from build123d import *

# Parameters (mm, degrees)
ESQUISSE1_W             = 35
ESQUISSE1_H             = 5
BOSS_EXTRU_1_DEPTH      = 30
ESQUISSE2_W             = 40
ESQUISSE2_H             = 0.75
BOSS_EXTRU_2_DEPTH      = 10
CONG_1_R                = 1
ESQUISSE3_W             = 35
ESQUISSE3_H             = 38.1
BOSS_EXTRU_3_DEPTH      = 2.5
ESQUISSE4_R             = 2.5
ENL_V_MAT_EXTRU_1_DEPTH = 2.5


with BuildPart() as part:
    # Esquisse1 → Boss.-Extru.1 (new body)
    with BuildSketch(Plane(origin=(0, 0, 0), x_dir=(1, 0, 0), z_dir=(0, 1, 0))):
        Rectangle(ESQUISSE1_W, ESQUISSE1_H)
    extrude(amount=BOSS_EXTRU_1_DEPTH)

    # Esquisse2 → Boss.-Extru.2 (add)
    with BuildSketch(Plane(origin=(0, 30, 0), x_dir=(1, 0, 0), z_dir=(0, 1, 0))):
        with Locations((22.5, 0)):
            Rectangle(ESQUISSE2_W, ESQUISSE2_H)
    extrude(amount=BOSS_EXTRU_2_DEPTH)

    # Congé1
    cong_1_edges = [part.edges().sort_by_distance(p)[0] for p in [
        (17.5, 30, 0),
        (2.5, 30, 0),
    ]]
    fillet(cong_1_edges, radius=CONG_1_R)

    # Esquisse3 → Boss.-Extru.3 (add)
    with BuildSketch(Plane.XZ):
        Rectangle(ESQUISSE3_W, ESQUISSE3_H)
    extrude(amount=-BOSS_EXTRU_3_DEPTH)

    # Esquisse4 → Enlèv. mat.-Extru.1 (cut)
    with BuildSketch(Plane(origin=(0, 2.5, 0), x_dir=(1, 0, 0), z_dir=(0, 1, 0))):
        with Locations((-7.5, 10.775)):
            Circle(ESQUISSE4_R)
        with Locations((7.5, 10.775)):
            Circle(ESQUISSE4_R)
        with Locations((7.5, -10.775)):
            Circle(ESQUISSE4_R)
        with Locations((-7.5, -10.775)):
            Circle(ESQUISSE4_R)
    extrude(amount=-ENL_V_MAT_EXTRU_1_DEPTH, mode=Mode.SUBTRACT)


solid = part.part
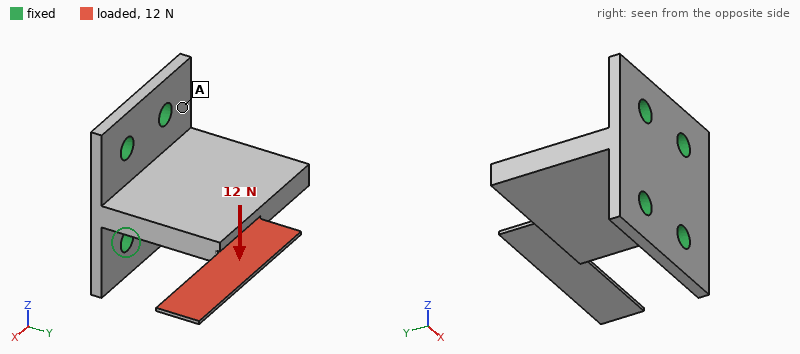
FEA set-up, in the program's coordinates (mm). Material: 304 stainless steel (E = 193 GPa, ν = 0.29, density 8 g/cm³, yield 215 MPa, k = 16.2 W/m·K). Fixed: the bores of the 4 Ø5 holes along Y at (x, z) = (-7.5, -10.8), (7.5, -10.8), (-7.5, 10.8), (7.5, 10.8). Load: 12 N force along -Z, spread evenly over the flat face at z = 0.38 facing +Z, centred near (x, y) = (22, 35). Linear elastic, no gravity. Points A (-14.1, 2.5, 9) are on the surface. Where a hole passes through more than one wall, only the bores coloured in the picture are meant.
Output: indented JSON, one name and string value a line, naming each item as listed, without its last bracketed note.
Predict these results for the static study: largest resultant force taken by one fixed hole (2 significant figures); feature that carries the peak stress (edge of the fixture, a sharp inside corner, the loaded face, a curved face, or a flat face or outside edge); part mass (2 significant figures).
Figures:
{
  "largest resultant force taken by one fixed hole": "20 N",
  "feature that carries the peak stress": "the loaded face",
  "part mass": "66 g"
}
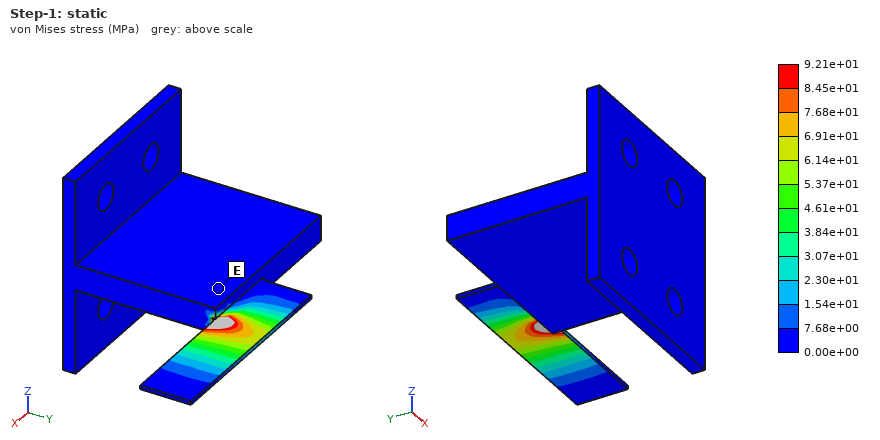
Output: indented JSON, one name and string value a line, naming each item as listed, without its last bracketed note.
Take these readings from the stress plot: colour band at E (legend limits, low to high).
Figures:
{
  "colour band at E": "0.00e+00 to 7.68e+00 MPa"
}
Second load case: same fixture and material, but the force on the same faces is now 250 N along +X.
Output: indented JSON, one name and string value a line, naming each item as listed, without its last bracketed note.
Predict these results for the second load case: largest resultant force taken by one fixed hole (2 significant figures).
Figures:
{
  "largest resultant force taken by one fixed hole": "230 N"
}
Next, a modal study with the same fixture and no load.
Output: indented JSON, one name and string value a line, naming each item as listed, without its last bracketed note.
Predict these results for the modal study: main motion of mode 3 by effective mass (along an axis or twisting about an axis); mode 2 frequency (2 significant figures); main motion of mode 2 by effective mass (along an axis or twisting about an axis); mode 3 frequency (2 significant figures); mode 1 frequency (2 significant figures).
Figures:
{
  "main motion of mode 3 by effective mass": "along Z",
  "mode 2 frequency": "3000 Hz",
  "main motion of mode 2 by effective mass": "along Z",
  "mode 3 frequency": "3700 Hz",
  "mode 1 frequency": "760 Hz"
}
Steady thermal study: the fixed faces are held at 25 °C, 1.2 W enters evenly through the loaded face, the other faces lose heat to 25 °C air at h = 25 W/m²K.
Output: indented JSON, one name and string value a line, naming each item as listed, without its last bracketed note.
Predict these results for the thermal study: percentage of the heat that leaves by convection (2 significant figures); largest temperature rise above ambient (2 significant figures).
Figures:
{
  "percentage of the heat that leaves by convection": "64 %",
  "largest temperature rise above ambient": "63 K"
}
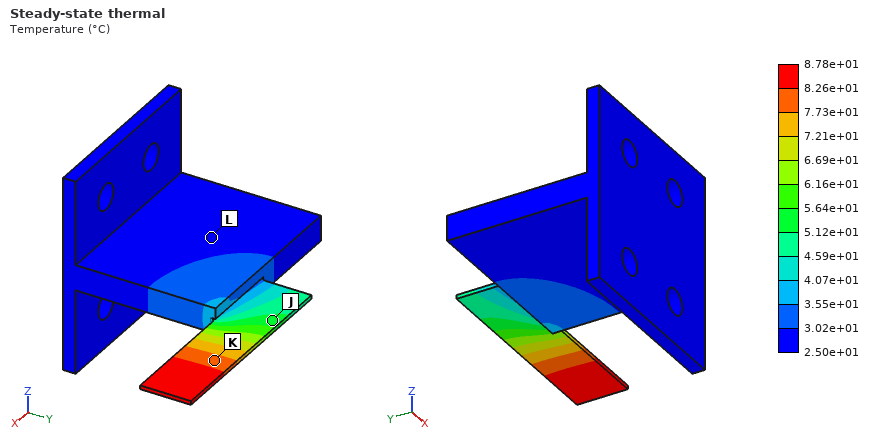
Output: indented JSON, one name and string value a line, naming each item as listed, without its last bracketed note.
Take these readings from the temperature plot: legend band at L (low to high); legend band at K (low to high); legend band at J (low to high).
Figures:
{
  "legend band at L": "2.50e+01 to 3.02e+01 °C",
  "legend band at K": "7.73e+01 to 8.26e+01 °C",
  "legend band at J": "5.12e+01 to 5.64e+01 °C"
}
